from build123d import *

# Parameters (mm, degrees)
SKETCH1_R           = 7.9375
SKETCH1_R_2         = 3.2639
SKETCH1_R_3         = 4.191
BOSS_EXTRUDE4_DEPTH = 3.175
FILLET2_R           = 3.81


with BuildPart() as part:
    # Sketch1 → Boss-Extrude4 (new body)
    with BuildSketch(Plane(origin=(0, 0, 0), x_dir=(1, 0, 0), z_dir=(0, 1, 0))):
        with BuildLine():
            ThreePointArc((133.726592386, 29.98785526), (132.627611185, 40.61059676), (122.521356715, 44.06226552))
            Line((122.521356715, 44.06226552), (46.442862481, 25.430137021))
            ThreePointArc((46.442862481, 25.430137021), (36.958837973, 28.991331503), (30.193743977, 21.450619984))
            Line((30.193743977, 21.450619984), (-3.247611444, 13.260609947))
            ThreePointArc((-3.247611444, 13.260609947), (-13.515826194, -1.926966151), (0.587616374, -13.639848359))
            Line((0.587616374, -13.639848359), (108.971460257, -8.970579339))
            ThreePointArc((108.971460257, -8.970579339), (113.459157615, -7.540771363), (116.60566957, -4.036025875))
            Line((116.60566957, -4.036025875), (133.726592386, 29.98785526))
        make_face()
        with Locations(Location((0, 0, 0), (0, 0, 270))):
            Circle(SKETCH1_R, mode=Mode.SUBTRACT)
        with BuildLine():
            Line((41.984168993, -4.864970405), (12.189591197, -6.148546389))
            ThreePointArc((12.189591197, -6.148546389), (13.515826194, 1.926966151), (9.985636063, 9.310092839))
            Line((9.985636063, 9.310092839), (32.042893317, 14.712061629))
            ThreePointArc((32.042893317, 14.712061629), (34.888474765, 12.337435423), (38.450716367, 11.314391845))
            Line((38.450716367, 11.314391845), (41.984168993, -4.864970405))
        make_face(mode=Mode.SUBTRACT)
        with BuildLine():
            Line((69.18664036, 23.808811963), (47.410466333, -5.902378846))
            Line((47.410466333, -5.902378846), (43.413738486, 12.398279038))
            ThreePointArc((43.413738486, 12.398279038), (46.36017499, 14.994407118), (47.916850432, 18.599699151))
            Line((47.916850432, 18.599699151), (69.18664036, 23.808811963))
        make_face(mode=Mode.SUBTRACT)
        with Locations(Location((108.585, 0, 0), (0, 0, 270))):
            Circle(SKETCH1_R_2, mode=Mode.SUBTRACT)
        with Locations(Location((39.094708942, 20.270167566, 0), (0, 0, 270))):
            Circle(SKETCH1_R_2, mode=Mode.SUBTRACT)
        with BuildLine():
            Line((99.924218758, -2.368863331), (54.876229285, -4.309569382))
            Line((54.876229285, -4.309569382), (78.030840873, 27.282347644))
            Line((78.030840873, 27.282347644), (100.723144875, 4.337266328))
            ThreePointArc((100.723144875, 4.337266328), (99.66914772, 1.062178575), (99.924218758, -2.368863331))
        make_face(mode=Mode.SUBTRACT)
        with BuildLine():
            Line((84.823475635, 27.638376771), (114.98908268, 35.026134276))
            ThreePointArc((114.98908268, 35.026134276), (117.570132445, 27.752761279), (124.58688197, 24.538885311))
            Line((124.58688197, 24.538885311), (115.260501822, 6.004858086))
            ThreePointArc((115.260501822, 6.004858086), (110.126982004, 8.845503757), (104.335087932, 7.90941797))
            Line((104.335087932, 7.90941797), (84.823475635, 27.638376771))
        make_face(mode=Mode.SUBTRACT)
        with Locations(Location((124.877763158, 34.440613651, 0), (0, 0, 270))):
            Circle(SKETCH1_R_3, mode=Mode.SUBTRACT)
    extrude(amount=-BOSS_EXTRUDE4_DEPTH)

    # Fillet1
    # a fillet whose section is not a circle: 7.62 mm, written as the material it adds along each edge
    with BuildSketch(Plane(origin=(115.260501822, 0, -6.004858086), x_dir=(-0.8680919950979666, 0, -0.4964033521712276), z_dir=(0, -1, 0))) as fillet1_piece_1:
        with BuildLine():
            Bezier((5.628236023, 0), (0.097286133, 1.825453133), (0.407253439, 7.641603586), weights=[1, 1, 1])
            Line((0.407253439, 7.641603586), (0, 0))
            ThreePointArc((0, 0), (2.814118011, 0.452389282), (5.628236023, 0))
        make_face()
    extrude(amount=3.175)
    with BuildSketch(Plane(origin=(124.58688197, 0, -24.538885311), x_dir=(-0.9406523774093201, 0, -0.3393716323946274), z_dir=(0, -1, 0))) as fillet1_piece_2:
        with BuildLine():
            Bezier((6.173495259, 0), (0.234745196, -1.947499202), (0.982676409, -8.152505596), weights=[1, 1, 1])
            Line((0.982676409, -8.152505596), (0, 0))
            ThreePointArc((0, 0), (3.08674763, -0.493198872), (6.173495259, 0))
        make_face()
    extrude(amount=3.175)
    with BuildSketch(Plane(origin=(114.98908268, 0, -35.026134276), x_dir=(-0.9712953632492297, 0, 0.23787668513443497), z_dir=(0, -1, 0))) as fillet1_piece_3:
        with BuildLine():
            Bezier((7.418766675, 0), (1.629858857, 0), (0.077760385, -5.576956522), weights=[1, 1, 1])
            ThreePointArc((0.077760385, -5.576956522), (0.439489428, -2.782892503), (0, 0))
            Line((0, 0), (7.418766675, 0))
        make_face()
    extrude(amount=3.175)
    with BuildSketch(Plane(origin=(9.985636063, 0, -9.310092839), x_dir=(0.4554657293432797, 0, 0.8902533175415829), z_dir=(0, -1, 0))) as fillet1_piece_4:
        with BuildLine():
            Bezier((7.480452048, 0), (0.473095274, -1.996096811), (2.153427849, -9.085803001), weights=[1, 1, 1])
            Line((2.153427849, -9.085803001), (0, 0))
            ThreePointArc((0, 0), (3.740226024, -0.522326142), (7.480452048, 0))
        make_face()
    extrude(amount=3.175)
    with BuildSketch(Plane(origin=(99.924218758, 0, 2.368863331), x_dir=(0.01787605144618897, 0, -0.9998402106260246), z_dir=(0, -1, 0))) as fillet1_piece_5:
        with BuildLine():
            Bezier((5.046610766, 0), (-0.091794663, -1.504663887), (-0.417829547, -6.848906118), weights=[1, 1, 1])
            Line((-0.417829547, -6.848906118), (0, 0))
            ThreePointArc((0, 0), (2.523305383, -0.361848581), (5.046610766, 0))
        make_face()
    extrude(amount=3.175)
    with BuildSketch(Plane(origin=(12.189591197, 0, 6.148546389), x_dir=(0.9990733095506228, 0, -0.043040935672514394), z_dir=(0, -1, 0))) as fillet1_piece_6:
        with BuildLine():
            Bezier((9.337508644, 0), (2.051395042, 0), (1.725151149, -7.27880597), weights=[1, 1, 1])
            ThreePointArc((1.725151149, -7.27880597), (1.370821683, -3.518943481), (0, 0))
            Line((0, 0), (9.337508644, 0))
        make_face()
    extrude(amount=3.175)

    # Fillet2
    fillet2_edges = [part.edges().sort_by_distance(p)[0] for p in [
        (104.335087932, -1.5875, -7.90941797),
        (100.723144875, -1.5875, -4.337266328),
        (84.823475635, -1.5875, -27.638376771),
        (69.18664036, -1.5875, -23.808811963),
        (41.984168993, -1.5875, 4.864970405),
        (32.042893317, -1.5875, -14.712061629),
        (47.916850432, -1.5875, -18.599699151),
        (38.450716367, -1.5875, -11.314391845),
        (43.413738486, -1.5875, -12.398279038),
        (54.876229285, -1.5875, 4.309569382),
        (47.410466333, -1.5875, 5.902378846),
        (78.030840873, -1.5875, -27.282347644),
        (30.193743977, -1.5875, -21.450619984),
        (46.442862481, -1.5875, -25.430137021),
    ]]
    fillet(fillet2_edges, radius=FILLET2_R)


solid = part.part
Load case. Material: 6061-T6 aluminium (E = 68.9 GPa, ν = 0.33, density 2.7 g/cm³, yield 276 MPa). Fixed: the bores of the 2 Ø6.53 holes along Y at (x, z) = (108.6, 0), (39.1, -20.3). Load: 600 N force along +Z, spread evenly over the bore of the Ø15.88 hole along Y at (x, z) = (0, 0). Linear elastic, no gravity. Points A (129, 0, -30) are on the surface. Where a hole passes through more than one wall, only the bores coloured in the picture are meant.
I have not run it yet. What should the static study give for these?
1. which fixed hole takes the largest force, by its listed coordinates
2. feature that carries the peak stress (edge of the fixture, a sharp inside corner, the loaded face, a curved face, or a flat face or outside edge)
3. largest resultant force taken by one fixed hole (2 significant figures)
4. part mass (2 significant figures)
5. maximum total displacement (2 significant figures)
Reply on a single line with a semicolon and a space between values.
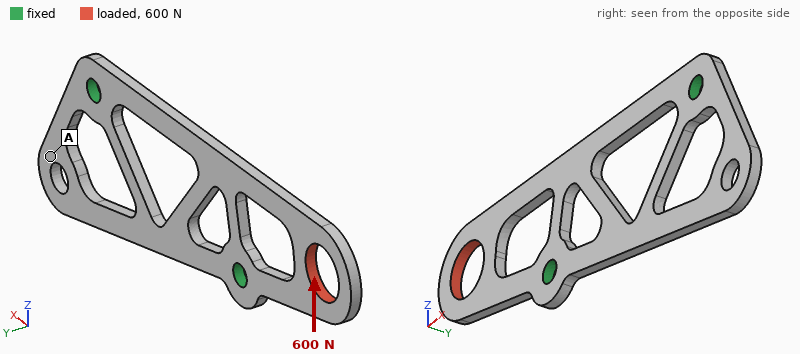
(39.1, -20.3); a curved face; 810 N; 27 g; 0.15 mm
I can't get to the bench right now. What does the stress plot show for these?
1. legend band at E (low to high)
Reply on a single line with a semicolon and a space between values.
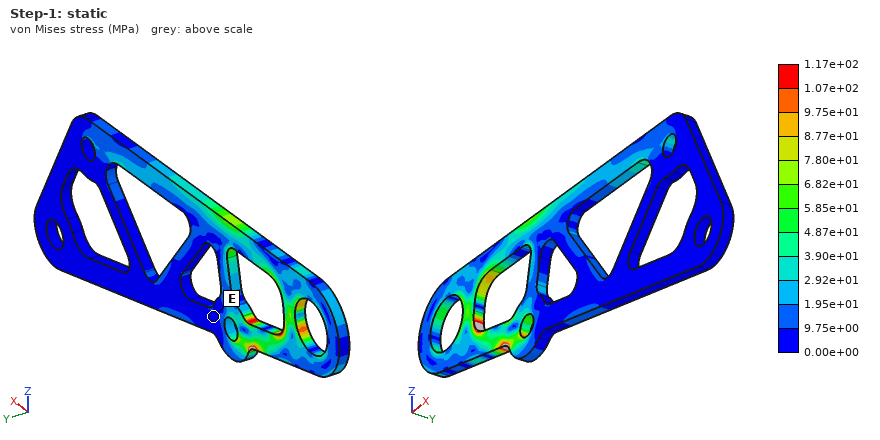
0.00e+00 to 9.75e+00 MPa
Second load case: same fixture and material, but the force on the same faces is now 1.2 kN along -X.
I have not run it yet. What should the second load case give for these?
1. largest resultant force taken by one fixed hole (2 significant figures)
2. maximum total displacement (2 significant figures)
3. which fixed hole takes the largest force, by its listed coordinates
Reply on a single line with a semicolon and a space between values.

730 N; 83 µm; (39.1, -20.3)
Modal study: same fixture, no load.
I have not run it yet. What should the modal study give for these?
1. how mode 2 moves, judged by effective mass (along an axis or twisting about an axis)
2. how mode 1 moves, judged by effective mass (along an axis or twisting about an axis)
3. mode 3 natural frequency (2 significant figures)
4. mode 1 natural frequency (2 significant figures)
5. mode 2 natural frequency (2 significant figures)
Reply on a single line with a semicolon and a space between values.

along Y; along Y; 1800 Hz; 770 Hz; 1000 Hz
